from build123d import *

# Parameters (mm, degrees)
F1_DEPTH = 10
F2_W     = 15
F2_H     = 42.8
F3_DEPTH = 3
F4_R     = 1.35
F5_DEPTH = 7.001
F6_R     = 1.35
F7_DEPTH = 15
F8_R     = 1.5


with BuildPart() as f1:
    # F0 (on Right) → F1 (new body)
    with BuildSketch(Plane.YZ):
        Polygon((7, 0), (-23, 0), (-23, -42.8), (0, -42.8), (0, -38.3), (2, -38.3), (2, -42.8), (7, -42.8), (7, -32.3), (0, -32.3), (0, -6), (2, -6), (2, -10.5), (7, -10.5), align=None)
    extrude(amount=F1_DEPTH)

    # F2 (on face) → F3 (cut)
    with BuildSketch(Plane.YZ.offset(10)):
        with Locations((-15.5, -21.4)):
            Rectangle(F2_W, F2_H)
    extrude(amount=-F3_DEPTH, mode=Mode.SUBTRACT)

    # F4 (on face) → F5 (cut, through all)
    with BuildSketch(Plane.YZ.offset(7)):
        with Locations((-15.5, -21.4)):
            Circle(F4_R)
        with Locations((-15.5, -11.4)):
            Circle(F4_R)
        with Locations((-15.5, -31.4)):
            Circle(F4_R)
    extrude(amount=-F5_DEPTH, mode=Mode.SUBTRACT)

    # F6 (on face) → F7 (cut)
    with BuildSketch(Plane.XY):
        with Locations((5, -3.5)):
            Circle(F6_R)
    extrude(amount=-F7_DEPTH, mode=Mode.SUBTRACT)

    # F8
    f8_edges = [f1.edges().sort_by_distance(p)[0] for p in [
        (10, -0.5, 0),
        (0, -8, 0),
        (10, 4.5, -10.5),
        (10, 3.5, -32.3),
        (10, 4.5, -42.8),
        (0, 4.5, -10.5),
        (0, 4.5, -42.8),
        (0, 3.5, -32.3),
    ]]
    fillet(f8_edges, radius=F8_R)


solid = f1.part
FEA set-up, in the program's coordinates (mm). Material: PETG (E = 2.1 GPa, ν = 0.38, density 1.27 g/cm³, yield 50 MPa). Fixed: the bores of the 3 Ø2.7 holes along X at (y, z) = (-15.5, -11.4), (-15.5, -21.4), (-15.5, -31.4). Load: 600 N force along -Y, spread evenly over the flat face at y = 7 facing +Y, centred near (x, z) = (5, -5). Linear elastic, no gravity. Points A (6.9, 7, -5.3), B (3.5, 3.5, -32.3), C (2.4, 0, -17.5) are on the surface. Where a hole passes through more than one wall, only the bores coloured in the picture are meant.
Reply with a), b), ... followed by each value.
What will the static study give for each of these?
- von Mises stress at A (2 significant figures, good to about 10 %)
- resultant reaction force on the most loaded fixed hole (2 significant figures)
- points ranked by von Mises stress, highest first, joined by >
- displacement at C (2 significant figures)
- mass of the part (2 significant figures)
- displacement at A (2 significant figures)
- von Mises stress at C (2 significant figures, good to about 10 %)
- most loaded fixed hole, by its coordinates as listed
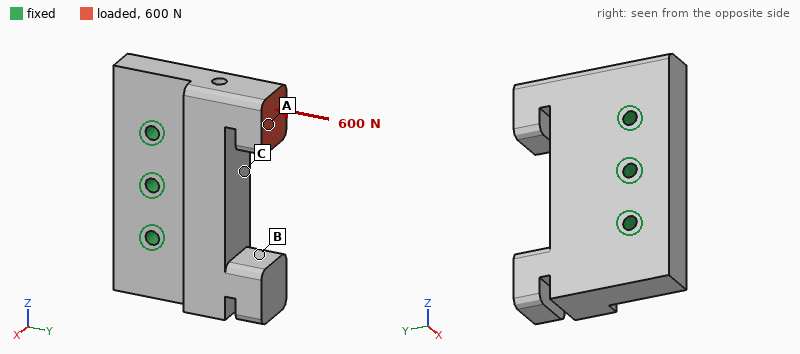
a) 14 MPa
b) 730 N
c) A > C > B
d) 0.067 mm
e) 11 g
f) 0.26 mm
g) 6.1 MPa
h) (-15.5, -11.4)
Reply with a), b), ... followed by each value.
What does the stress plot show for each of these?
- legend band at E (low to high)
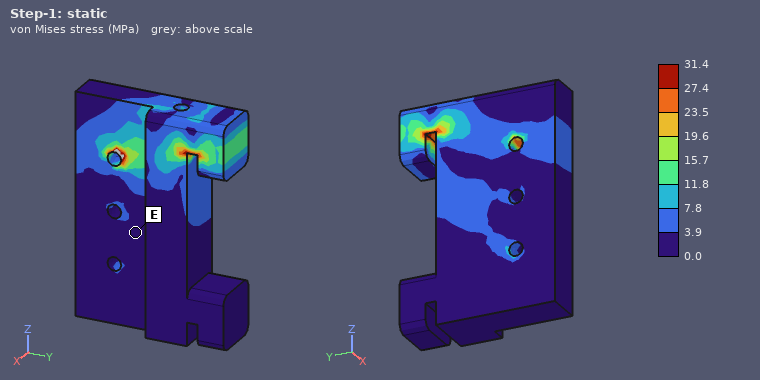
a) 0.0 to 3.9 MPa
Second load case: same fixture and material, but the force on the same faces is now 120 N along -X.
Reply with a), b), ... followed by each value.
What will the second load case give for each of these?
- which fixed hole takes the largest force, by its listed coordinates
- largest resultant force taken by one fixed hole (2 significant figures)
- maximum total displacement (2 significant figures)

a) (-15.5, -11.4)
b) 110 N
c) 0.52 mm
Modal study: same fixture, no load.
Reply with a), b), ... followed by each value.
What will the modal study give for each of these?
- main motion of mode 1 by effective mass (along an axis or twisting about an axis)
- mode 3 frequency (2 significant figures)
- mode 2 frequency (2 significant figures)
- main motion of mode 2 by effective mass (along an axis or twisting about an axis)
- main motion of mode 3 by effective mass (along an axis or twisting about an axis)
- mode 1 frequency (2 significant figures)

a) along X
b) 4400 Hz
c) 2900 Hz
d) twisting about Y
e) along Z
f) 2600 Hz
